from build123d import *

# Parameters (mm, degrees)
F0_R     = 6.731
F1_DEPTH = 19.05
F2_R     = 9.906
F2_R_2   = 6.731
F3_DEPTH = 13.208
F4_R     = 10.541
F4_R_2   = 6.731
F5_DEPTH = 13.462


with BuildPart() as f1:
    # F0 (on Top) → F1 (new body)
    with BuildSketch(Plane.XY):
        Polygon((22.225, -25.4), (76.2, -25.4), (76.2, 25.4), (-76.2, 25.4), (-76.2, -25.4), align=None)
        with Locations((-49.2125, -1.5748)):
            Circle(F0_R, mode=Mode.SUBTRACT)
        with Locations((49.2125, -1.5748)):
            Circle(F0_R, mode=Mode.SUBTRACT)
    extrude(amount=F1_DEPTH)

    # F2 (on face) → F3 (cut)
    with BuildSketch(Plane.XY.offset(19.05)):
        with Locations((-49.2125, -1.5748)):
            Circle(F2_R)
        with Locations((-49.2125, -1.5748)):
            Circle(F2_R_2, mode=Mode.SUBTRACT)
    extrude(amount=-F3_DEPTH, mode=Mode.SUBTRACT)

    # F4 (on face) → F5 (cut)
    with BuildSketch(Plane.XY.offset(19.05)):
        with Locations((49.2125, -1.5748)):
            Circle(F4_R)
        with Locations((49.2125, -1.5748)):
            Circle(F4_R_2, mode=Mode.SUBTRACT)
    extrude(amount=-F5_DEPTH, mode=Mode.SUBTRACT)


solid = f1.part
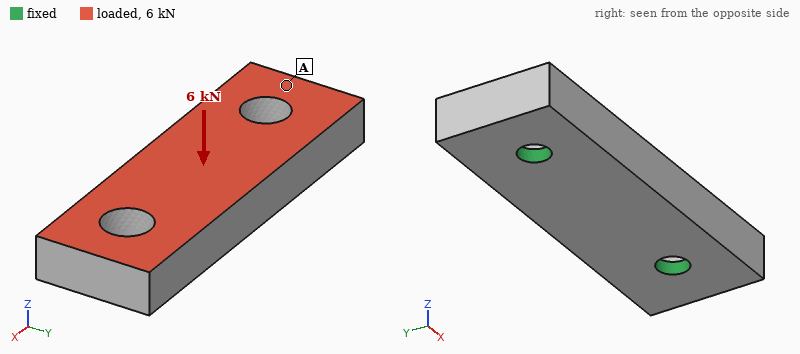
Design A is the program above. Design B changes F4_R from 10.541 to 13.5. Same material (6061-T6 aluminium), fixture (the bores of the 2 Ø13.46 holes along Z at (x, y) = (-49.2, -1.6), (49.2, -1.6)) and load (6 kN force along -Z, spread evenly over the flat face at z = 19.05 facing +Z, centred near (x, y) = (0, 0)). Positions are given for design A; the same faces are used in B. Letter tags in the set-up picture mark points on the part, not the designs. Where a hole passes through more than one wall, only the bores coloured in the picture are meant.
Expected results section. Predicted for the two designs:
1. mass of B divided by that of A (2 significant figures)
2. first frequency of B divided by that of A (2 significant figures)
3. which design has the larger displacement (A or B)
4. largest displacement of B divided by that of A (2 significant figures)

0.98
0.96
B
1.1
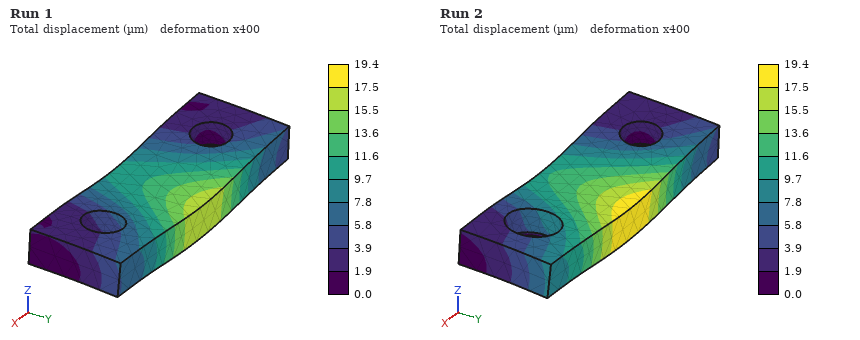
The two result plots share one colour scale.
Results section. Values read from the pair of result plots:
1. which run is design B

Run 2
